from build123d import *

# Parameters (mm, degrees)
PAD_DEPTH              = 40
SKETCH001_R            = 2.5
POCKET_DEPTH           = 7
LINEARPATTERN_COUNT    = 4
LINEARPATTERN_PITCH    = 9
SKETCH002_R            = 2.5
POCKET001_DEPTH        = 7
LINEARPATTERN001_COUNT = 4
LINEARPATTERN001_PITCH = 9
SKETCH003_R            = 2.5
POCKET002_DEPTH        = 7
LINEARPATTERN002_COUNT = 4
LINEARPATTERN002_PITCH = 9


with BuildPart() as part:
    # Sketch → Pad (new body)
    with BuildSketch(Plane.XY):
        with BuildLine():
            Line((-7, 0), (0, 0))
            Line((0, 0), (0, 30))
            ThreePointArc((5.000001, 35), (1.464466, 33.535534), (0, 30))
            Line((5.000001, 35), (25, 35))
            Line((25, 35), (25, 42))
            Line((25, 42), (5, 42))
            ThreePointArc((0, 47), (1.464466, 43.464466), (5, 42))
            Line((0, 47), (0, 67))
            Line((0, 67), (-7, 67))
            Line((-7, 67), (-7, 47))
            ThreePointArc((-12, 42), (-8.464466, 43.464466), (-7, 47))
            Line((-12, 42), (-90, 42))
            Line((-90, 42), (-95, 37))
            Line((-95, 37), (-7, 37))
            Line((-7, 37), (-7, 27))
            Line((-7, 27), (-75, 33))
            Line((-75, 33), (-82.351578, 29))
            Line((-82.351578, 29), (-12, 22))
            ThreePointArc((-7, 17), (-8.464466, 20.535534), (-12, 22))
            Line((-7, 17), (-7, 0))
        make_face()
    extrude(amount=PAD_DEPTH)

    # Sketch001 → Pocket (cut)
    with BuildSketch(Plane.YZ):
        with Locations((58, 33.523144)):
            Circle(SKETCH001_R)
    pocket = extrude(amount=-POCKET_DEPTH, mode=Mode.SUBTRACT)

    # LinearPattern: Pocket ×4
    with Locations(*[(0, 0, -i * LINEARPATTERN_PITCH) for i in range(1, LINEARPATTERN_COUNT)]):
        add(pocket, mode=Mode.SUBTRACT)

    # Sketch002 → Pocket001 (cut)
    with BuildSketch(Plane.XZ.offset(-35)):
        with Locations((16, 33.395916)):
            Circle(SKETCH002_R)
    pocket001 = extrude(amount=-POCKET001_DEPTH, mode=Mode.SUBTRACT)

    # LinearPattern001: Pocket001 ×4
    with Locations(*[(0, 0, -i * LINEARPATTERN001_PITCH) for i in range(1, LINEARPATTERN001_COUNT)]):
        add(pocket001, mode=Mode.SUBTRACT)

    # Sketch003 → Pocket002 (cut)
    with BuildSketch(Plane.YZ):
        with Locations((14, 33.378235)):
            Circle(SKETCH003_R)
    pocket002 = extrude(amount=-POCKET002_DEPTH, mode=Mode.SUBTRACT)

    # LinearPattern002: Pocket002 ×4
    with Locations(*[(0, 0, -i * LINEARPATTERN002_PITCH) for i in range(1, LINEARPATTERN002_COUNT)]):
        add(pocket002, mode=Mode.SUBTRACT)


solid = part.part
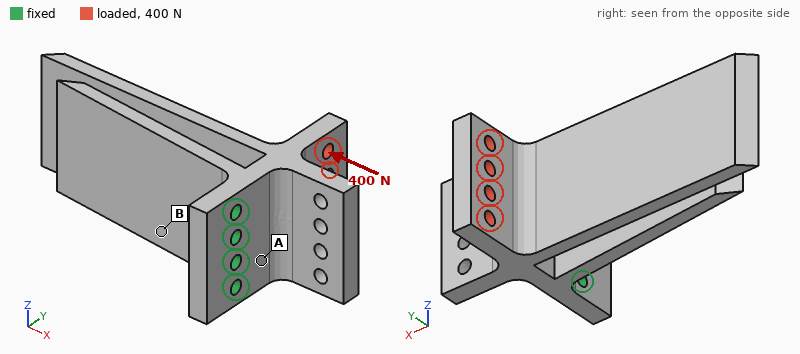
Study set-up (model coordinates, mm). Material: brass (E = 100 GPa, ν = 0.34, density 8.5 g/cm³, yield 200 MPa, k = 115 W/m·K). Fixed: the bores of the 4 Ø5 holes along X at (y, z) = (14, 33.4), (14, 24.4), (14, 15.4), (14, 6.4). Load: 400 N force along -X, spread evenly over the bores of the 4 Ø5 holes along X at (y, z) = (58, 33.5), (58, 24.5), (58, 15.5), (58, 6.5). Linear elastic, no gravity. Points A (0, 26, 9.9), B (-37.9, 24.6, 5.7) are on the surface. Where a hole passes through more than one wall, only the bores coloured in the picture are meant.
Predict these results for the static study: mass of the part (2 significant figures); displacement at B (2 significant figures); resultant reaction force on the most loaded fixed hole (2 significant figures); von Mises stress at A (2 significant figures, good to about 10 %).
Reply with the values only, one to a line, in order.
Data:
480 g
0.028 mm
120 N
30 MPa
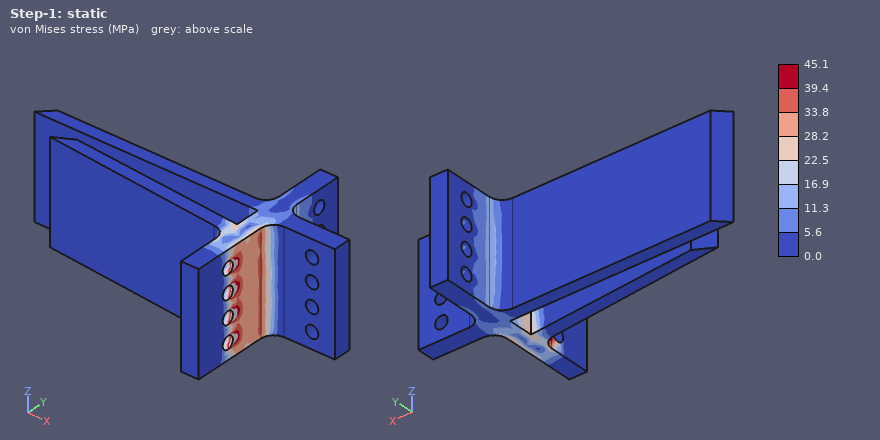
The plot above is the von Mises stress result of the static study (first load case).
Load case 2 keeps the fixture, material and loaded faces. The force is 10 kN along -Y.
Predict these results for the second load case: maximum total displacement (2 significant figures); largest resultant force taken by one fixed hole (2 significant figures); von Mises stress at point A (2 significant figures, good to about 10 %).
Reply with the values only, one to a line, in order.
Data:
17 µm
2.9 kN
39 MPa
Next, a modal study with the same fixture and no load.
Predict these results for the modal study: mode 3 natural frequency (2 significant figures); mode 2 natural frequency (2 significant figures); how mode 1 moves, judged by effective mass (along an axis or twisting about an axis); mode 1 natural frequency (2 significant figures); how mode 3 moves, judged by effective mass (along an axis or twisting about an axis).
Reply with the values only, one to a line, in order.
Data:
990 Hz
560 Hz
along Y
330 Hz
along Z
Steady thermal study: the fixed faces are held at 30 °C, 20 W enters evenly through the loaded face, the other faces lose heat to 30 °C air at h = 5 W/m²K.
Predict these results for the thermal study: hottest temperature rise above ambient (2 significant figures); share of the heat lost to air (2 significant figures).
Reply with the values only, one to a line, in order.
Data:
25 K
5.4 %
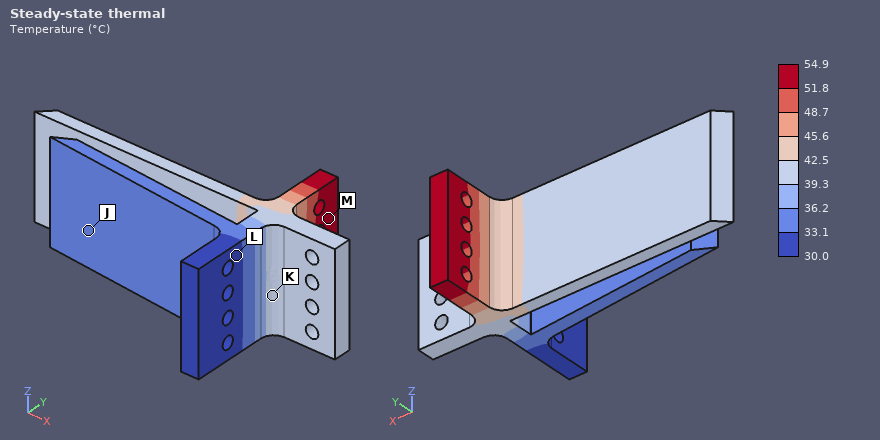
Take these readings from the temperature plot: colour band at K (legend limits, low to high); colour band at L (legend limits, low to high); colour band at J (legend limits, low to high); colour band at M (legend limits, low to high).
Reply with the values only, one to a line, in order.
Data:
39.3 to 42.5 °C
30.0 to 33.1 °C
33.1 to 36.2 °C
51.8 to 54.9 °C
